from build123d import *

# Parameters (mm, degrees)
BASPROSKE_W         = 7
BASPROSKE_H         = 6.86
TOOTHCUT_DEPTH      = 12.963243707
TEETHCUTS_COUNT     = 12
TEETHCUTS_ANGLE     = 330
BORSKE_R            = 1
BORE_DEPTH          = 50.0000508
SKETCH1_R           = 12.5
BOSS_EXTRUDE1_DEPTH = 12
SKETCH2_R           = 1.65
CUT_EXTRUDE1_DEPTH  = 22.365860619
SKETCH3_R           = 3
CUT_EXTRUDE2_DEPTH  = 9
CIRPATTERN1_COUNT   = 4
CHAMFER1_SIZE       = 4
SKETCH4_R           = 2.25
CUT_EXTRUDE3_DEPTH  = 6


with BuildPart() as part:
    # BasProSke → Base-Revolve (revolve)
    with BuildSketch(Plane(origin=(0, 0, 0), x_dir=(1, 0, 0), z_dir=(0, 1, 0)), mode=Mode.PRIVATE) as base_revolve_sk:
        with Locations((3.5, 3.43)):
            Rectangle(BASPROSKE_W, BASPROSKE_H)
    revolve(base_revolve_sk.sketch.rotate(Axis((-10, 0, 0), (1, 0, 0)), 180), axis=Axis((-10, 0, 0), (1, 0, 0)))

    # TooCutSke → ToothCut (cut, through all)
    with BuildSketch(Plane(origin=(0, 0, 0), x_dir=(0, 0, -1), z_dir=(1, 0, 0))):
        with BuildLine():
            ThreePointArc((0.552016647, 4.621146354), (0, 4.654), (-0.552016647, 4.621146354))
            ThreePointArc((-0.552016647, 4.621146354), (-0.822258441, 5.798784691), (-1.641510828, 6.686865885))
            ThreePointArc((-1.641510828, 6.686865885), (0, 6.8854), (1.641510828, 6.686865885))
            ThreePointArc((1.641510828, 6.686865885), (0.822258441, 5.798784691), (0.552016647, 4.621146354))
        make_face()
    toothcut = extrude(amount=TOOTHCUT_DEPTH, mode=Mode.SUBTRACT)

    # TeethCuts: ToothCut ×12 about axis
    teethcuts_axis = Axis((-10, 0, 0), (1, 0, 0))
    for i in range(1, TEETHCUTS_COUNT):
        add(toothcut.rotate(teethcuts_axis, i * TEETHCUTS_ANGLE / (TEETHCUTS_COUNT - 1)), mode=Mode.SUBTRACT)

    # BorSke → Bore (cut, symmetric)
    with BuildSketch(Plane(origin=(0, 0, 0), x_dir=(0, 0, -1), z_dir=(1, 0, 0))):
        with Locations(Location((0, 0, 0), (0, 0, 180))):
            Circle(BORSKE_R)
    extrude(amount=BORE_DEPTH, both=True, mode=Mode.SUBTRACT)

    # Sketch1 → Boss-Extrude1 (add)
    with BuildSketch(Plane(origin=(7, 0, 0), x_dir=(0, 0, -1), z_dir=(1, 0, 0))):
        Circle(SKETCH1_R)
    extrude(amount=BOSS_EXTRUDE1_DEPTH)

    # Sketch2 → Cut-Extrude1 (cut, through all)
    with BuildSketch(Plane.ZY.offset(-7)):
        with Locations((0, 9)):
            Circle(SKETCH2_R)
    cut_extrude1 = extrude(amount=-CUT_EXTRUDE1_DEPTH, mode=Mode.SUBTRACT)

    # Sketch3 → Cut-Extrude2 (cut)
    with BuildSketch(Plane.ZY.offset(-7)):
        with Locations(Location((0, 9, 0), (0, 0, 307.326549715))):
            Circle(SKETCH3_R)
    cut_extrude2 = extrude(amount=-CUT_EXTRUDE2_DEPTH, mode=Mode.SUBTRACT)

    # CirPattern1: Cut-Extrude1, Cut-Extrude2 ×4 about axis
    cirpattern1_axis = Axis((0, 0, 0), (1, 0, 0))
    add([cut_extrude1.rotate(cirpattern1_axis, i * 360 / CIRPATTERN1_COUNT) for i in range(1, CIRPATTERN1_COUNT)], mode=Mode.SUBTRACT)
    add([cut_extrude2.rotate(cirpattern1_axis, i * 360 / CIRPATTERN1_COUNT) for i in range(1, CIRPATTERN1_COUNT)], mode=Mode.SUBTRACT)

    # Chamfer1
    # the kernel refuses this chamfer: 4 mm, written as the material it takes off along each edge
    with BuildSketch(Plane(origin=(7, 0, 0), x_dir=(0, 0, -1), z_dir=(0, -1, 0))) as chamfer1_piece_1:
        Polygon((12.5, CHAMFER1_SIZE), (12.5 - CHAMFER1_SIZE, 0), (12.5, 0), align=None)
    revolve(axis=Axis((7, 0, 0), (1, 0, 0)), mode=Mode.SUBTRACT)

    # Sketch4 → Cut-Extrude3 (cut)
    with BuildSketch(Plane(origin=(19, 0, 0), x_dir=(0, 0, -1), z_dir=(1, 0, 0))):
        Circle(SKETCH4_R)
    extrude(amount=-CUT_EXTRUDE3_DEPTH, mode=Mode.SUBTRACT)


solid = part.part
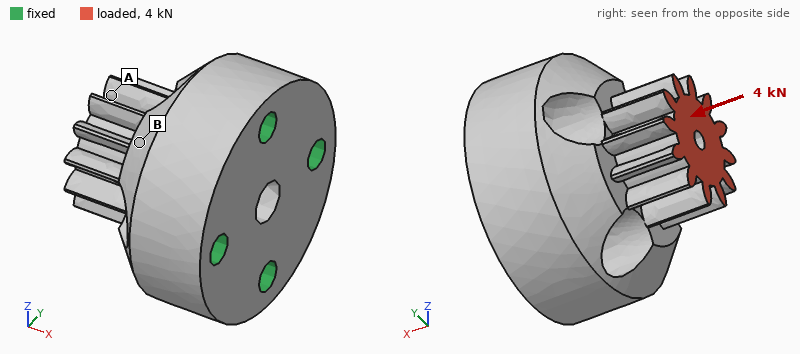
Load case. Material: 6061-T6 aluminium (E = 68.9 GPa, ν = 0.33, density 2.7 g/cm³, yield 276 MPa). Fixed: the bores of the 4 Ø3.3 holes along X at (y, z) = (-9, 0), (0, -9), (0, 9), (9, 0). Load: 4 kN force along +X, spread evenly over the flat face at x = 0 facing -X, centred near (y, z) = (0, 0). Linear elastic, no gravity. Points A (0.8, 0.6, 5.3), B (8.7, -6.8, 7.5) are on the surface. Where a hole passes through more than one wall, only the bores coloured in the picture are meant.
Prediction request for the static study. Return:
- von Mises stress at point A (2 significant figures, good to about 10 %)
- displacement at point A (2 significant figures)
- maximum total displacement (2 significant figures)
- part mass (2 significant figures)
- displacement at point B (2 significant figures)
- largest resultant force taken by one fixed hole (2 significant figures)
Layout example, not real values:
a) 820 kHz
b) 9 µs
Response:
a) 41 MPa
b) 10 µm
c) 11 µm
d) 13 g
e) 3.4 µm
f) 1.1 kN
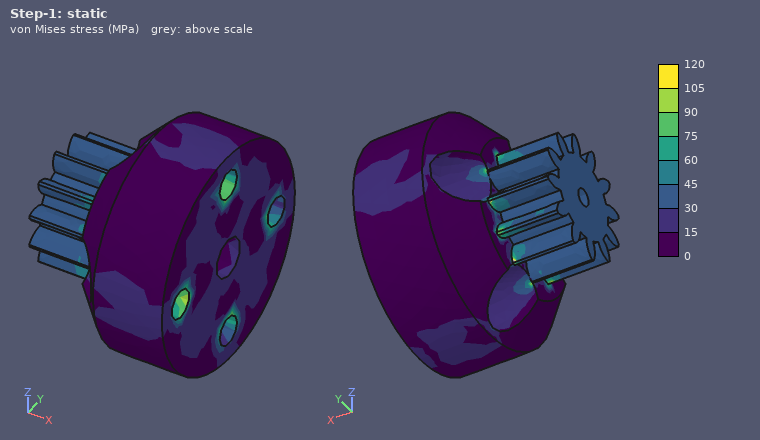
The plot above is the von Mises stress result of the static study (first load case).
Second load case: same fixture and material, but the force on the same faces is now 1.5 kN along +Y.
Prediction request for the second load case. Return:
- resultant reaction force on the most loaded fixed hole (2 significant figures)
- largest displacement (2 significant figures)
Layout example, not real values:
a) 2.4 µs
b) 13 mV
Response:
a) 1.4 kN
b) 30 µm
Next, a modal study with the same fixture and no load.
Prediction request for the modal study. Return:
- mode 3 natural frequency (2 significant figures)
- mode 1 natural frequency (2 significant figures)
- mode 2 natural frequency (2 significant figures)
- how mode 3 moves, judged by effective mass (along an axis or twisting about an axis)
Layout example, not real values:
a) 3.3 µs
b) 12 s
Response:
a) 48 kHz
b) 29 kHz
c) 29 kHz
d) along X
